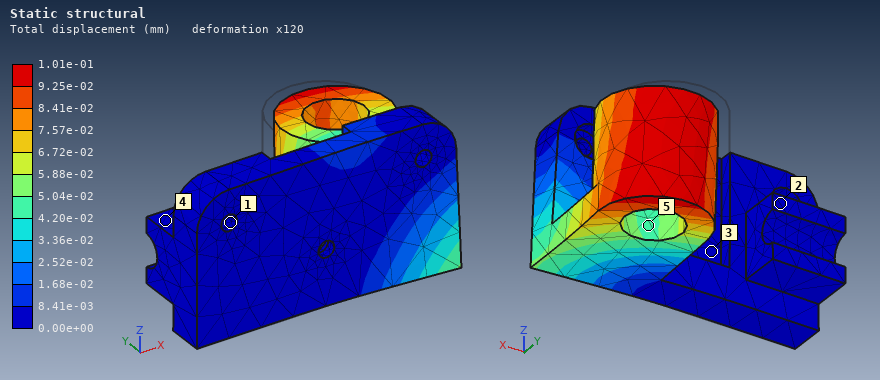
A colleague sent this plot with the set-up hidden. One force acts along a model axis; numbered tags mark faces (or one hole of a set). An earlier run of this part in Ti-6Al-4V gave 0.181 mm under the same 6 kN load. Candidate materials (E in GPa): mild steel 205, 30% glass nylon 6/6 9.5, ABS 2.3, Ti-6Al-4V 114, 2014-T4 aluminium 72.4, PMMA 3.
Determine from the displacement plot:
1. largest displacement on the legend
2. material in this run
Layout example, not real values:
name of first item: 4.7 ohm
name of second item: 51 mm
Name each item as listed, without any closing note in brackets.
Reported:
largest displacement on the legend: 1.01e-01 mm
material in this run: mild steel
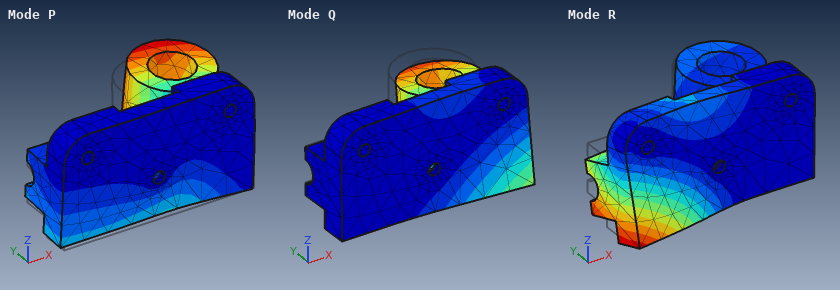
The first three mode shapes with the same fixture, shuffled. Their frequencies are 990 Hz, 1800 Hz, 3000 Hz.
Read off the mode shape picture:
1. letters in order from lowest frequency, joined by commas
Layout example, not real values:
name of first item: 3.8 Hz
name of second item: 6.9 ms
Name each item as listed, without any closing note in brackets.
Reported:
letters in order from lowest frequency, joined by commas: Q, P, R
